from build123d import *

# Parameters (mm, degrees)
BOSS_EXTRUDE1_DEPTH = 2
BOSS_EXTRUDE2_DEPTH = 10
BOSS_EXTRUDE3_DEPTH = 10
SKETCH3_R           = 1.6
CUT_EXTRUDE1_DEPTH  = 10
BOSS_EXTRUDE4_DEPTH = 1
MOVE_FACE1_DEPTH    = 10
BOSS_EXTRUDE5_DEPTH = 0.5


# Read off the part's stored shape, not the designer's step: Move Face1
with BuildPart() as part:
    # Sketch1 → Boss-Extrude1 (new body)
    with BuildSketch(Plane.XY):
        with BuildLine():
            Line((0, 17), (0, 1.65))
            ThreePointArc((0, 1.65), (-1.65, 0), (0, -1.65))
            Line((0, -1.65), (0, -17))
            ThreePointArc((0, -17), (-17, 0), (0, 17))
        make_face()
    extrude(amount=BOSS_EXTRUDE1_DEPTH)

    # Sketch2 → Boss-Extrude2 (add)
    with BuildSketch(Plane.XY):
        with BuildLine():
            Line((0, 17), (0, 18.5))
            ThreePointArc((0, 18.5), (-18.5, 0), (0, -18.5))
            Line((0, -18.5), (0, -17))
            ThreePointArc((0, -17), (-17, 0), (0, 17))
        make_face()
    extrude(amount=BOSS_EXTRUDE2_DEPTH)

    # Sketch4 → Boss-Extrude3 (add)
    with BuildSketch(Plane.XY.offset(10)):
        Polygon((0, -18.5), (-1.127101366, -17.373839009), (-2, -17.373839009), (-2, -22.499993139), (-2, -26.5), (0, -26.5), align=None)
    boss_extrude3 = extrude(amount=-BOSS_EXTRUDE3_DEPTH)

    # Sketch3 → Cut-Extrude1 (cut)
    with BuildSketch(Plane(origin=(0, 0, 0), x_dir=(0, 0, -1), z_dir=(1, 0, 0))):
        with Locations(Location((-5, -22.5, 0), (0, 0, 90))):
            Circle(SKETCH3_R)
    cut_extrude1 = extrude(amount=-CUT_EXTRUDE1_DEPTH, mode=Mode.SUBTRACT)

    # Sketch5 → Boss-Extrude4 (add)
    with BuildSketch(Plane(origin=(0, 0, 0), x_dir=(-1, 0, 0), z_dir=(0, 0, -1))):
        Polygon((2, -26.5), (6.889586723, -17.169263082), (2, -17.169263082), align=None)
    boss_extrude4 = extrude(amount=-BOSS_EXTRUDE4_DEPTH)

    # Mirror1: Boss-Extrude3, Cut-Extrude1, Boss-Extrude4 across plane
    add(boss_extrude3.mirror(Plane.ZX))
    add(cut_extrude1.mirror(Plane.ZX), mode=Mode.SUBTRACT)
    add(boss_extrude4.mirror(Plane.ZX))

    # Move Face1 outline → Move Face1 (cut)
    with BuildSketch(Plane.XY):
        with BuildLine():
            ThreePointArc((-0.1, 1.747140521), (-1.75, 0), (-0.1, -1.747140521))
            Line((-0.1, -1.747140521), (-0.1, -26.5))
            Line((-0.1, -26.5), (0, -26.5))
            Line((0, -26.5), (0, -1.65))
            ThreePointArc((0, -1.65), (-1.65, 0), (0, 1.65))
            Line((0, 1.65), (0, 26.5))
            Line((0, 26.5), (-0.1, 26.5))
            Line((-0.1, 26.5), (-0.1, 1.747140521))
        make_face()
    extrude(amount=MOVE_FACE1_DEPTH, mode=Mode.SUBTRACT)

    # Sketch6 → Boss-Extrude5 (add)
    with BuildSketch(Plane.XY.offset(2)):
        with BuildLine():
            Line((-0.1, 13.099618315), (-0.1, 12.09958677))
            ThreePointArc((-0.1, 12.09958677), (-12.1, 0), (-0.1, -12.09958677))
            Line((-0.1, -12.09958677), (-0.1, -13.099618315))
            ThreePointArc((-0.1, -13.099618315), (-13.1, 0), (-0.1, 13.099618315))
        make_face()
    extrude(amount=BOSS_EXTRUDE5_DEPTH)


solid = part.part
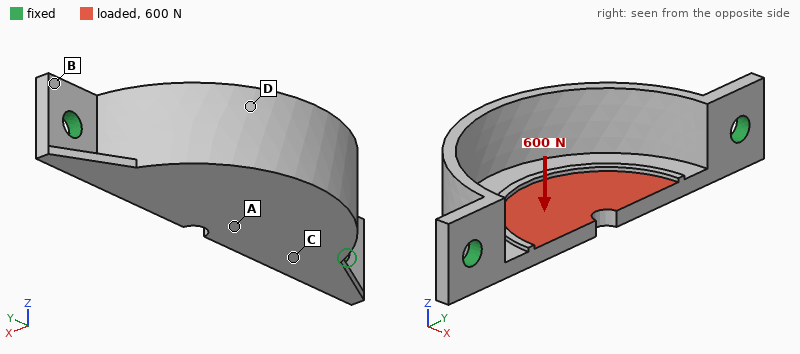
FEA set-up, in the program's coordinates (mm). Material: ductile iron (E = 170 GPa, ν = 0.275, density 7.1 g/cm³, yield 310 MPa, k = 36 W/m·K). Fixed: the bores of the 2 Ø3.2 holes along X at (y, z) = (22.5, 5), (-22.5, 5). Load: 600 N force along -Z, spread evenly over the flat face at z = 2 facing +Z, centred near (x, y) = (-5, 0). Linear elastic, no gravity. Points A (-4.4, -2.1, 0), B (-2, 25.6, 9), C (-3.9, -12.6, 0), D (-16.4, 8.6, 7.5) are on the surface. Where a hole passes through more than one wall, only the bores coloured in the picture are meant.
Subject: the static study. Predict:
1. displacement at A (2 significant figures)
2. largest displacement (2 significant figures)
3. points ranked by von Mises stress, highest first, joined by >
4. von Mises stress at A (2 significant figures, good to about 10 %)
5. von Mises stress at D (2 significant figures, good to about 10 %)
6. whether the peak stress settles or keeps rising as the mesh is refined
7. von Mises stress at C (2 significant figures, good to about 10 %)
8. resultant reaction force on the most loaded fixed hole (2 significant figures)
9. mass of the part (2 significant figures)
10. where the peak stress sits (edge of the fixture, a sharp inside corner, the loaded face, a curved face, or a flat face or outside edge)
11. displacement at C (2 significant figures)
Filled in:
63 µm
74 µm
A > C > D > B
120 MPa
36 MPa
keeps rising
91 MPa
350 N
15 g
edge of the fixture
26 µm
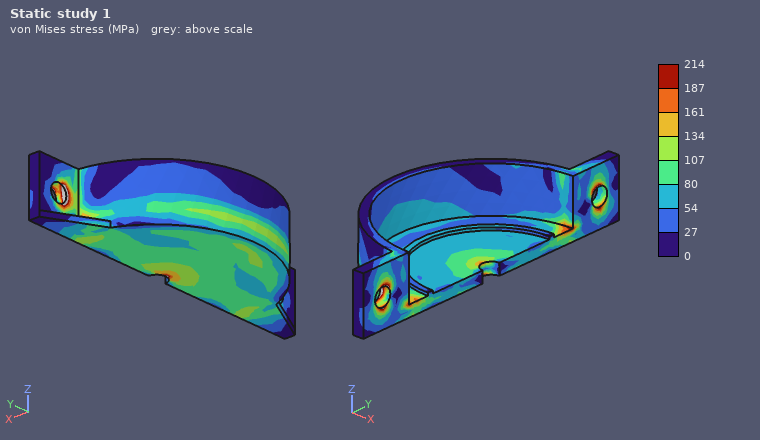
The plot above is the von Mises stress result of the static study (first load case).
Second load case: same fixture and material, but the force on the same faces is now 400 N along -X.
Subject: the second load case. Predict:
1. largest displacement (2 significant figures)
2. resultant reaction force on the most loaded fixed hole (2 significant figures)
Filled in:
17 µm
250 N
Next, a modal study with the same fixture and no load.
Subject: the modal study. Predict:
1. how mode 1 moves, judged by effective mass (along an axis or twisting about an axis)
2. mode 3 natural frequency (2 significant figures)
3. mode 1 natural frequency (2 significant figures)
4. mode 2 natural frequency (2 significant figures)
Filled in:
along Z
10 kHz
4500 Hz
10 kHz
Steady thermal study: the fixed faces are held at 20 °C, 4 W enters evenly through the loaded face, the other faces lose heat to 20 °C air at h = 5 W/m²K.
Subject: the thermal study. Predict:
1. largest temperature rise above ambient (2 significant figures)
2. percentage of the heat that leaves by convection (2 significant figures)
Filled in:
42 K
7.1 %
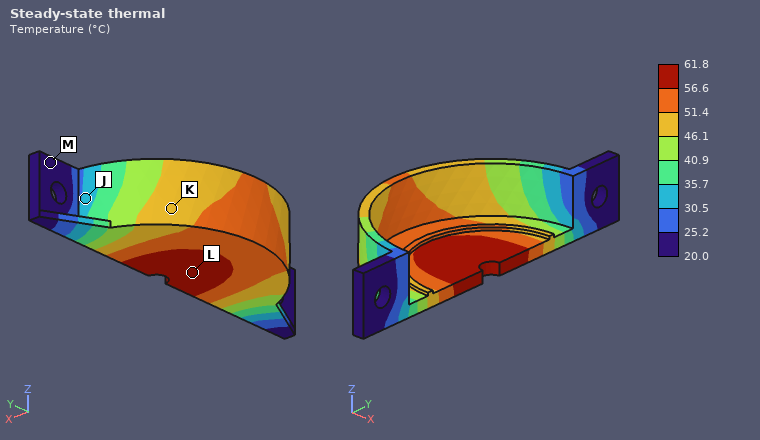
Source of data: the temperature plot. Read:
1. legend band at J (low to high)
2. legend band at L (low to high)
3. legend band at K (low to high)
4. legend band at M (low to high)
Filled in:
30.5 to 35.7 °C
56.6 to 61.8 °C
46.1 to 51.4 °C
20.0 to 25.2 °C
